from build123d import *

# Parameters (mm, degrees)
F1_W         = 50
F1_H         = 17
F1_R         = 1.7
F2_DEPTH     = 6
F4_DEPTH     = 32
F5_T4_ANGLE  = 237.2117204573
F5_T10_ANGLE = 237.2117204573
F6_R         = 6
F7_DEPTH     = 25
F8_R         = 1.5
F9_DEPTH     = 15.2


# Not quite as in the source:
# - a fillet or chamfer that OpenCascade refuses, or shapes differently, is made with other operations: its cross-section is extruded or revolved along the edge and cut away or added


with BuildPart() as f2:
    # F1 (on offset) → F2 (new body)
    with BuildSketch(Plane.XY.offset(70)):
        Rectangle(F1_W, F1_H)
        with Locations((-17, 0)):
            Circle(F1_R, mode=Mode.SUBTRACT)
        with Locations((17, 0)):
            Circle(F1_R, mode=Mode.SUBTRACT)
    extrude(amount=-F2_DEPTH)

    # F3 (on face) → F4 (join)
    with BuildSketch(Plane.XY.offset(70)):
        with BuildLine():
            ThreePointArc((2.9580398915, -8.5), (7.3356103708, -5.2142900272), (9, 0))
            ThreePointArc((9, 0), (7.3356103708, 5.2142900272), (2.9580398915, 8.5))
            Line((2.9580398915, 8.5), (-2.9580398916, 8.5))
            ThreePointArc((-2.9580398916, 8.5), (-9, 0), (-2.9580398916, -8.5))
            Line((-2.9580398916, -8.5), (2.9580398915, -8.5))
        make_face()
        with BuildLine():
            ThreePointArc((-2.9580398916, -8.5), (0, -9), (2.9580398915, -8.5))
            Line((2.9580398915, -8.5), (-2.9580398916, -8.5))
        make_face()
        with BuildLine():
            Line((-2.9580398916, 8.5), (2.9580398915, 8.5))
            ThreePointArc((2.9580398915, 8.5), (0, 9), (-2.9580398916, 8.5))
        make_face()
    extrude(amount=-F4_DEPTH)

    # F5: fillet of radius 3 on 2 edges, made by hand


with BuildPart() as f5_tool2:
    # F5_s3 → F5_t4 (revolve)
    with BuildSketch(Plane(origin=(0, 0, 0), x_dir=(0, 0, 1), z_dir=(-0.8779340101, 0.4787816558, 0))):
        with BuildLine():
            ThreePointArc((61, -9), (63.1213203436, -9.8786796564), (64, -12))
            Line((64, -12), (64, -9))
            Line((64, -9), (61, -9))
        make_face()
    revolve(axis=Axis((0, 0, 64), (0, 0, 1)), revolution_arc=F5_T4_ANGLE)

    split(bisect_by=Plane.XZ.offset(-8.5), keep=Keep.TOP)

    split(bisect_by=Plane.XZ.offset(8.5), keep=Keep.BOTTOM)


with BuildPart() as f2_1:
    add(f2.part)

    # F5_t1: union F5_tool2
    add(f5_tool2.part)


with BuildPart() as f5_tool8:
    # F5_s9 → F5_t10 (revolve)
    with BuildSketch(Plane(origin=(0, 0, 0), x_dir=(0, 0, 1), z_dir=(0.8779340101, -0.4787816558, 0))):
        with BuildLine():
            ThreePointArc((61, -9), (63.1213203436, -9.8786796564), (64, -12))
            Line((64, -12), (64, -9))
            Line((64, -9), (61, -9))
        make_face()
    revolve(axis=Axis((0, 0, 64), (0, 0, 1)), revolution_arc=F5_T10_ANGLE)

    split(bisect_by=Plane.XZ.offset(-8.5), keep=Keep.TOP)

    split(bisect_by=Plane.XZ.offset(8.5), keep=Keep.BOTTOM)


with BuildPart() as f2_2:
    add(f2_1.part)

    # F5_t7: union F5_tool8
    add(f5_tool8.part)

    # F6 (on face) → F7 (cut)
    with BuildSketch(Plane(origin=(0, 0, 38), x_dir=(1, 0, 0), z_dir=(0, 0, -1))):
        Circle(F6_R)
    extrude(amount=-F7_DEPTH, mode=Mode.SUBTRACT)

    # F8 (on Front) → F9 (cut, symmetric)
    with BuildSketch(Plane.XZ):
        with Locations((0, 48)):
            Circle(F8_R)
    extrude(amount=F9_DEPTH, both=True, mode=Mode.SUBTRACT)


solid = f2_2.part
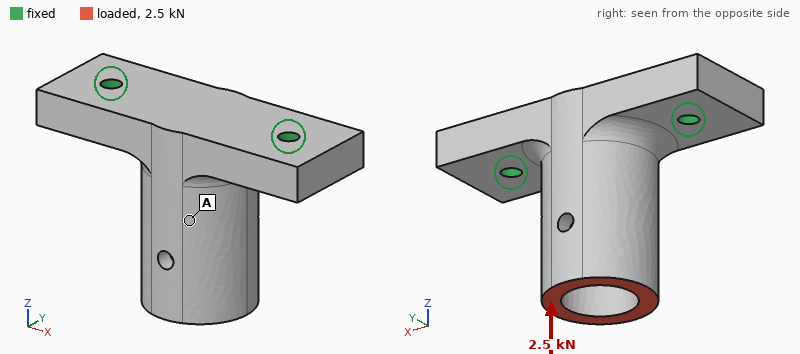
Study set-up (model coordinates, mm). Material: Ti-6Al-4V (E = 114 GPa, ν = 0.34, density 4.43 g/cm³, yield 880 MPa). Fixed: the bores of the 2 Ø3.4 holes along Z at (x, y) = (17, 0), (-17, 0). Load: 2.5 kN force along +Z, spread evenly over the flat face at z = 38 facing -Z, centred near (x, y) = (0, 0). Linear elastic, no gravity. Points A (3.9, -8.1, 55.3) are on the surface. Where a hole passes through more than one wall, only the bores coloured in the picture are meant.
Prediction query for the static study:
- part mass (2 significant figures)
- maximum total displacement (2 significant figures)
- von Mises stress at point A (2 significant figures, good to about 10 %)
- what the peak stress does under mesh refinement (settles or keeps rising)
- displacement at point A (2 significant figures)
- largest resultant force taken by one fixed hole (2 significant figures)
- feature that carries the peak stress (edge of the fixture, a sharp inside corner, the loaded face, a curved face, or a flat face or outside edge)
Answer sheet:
39 g
13 µm
11 MPa
keeps rising
10 µm
1.3 kN
edge of the fixture
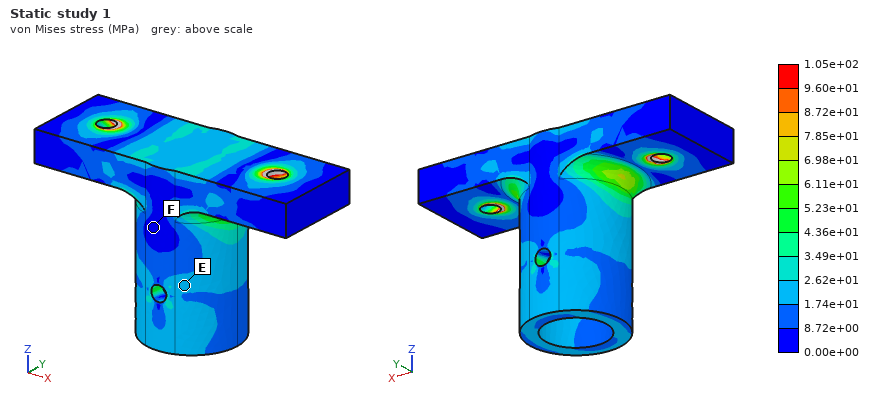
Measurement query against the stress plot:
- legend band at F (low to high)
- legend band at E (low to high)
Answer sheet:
0.00e+00 to 8.72e+00 MPa
1.74e+01 to 2.62e+01 MPa
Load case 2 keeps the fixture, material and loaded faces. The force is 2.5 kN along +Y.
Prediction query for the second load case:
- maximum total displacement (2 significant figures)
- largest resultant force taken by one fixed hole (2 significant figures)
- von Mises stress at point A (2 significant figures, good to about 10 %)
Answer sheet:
0.31 mm
1.3 kN
86 MPa
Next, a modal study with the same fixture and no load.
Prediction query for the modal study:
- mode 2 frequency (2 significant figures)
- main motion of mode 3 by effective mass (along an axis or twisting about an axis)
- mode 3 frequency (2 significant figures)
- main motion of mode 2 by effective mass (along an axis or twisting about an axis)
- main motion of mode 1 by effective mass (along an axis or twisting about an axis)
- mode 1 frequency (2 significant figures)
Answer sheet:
12 kHz
along Z
16 kHz
along X
along Y
5700 Hz
